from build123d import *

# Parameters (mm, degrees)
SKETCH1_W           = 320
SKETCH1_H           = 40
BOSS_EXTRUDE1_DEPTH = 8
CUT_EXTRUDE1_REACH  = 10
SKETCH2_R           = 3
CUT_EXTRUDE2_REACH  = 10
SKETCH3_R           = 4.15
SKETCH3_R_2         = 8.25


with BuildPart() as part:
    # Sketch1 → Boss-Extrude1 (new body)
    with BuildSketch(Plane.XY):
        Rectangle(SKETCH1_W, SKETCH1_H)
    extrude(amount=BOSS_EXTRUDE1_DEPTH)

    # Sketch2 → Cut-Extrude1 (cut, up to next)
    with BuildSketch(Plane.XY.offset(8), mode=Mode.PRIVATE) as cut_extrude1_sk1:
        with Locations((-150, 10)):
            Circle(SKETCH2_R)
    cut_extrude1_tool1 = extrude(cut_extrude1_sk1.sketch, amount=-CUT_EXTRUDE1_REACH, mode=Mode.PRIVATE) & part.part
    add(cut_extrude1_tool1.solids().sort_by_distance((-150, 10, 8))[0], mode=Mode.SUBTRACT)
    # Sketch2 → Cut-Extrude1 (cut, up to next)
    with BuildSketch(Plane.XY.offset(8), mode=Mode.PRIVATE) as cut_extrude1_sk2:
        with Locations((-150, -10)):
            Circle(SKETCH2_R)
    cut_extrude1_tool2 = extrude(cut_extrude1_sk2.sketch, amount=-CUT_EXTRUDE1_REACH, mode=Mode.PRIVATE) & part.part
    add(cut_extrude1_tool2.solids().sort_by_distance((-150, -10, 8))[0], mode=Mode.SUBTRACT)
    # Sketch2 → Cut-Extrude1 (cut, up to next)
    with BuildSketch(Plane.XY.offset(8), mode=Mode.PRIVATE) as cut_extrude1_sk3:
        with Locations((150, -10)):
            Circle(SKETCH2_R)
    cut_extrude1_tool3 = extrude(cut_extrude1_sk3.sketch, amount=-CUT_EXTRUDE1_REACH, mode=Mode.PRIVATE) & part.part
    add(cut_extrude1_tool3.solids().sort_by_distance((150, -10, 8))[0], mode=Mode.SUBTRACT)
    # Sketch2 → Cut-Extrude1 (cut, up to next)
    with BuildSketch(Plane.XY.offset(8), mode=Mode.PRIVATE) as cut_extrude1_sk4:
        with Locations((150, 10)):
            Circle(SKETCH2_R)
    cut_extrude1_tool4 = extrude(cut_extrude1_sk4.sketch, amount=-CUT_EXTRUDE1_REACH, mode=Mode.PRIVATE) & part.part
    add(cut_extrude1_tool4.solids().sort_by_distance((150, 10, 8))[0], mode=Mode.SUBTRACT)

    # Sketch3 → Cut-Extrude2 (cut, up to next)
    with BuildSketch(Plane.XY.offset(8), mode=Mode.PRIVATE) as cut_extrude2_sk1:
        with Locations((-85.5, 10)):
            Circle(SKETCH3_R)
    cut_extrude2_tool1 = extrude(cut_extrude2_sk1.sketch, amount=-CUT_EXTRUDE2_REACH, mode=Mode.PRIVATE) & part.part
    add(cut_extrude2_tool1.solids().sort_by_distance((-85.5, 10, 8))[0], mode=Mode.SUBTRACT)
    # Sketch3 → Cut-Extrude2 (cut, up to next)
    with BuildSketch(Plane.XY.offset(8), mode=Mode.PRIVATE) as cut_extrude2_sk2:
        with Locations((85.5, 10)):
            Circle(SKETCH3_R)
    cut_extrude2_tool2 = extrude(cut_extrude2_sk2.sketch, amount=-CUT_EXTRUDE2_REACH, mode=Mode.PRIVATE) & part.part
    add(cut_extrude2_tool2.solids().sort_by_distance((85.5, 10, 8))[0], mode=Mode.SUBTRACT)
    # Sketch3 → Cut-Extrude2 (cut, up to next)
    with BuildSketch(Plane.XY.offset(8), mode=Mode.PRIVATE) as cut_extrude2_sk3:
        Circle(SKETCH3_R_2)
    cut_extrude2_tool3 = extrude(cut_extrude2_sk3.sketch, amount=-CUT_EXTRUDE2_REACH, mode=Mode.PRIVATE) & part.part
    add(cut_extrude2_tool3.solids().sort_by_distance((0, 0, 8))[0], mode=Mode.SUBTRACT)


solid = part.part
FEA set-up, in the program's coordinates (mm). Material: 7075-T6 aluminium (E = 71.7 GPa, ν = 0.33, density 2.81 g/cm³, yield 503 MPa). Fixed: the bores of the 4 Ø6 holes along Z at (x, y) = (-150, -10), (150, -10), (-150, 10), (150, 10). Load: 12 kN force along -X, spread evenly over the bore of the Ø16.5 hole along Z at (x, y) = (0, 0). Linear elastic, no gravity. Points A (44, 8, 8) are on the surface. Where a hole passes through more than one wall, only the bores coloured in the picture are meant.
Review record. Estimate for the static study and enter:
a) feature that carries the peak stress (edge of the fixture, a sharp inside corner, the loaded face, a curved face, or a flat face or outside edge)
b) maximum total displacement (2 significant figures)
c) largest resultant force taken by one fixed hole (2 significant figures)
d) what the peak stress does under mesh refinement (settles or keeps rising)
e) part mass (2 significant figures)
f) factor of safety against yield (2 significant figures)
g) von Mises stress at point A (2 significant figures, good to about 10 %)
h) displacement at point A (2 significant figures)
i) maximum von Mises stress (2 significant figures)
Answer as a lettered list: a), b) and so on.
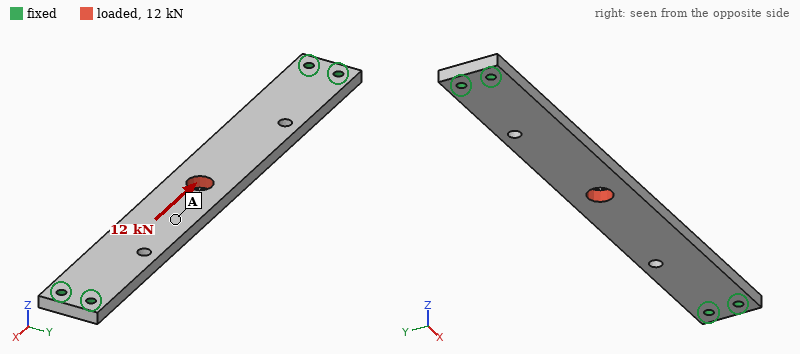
a) a curved face
b) 42 µm
c) 3.1 kN
d) settles
e) 280 g
f) 8.2
g) 19 MPa
h) 29 µm
i) 61 MPa
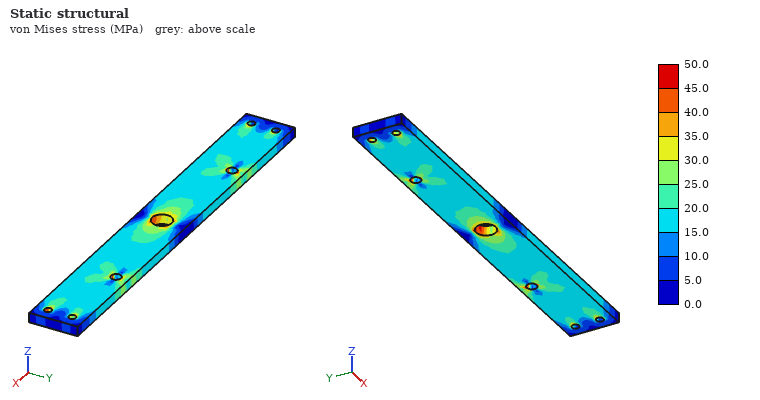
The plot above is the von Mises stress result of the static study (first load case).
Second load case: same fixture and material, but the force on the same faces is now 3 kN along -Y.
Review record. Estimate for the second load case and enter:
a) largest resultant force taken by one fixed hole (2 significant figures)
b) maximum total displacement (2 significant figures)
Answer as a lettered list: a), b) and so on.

a) 4.6 kN
b) 0.18 mm
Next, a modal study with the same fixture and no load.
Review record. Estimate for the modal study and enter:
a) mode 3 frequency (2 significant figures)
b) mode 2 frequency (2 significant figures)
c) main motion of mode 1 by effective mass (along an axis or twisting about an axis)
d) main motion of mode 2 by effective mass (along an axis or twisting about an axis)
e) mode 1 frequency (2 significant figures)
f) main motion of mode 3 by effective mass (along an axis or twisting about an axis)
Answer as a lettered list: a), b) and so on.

a) 2000 Hz
b) 1300 Hz
c) along Z
d) twisting about Y
e) 470 Hz
f) twisting about X
